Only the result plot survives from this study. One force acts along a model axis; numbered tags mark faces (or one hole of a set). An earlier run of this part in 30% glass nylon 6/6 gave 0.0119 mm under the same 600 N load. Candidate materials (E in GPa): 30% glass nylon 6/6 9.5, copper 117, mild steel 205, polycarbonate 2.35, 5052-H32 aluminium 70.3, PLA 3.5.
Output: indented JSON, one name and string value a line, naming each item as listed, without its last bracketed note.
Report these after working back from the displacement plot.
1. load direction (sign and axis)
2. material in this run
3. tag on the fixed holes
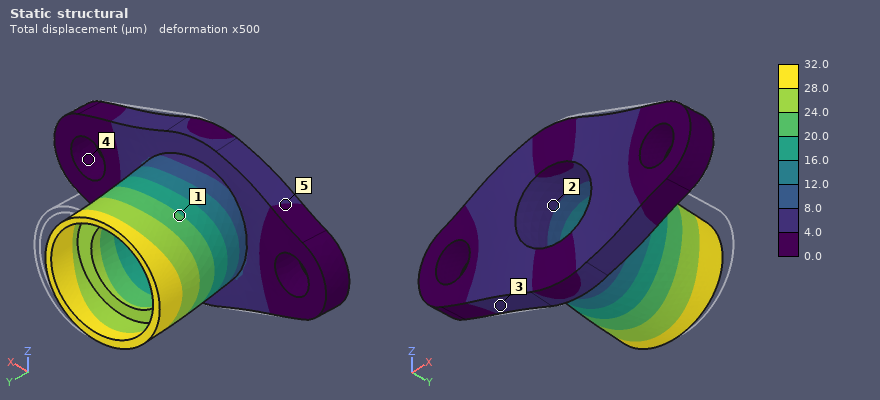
{
  "load direction": "-X",
  "material in this run": "PLA",
  "tag on the fixed holes": "4"
}
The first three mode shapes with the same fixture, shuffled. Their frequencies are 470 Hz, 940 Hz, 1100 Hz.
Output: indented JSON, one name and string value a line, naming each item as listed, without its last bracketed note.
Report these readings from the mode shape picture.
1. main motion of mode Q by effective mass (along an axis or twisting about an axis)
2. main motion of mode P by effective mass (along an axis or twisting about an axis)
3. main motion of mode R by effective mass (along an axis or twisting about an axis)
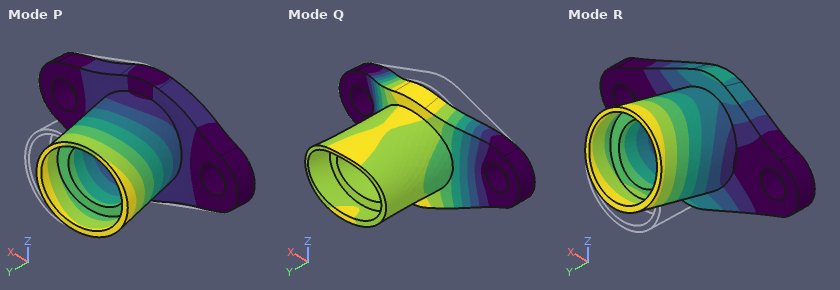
{
  "main motion of mode Q by effective mass": "along Y",
  "main motion of mode P by effective mass": "along X",
  "main motion of mode R by effective mass": "along Z"
}
